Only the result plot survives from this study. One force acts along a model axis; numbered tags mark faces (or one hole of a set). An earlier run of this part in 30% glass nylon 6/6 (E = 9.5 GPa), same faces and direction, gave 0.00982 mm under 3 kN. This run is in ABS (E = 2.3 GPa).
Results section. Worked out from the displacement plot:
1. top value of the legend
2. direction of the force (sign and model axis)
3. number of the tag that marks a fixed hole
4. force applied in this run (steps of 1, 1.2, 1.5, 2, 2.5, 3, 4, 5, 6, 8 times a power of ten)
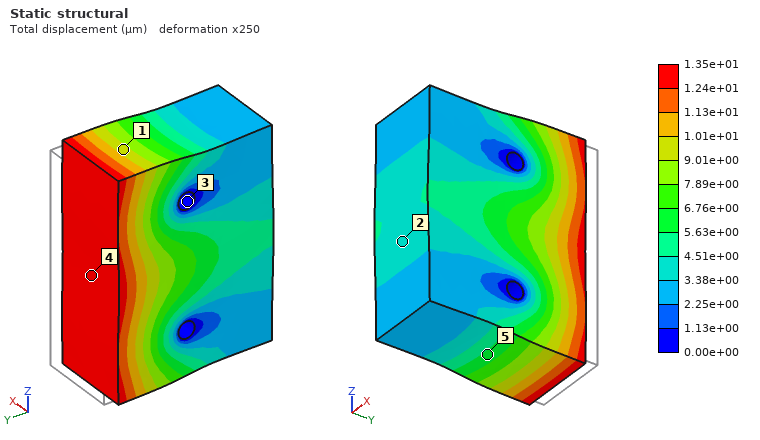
1.35e+01 µm
-Y
3
1 kN
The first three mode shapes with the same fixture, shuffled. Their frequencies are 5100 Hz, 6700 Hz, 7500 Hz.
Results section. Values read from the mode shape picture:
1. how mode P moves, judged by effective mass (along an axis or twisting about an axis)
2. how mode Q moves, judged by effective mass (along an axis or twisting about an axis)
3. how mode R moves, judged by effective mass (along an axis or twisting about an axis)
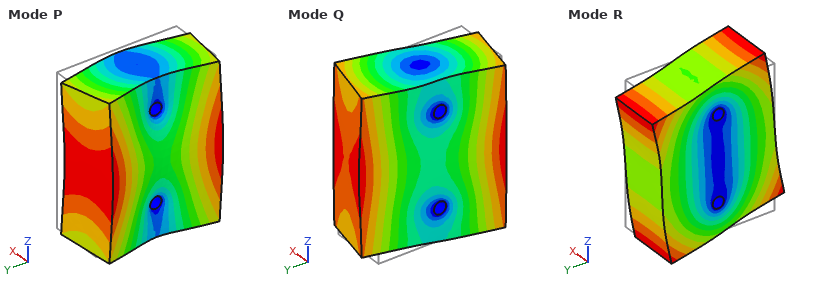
along X
twisting about Z
twisting about X
